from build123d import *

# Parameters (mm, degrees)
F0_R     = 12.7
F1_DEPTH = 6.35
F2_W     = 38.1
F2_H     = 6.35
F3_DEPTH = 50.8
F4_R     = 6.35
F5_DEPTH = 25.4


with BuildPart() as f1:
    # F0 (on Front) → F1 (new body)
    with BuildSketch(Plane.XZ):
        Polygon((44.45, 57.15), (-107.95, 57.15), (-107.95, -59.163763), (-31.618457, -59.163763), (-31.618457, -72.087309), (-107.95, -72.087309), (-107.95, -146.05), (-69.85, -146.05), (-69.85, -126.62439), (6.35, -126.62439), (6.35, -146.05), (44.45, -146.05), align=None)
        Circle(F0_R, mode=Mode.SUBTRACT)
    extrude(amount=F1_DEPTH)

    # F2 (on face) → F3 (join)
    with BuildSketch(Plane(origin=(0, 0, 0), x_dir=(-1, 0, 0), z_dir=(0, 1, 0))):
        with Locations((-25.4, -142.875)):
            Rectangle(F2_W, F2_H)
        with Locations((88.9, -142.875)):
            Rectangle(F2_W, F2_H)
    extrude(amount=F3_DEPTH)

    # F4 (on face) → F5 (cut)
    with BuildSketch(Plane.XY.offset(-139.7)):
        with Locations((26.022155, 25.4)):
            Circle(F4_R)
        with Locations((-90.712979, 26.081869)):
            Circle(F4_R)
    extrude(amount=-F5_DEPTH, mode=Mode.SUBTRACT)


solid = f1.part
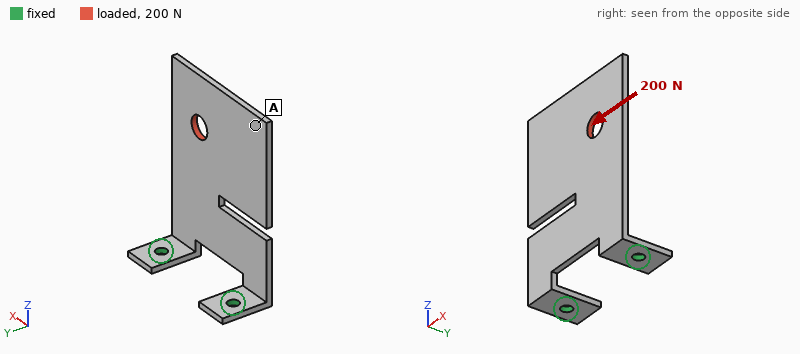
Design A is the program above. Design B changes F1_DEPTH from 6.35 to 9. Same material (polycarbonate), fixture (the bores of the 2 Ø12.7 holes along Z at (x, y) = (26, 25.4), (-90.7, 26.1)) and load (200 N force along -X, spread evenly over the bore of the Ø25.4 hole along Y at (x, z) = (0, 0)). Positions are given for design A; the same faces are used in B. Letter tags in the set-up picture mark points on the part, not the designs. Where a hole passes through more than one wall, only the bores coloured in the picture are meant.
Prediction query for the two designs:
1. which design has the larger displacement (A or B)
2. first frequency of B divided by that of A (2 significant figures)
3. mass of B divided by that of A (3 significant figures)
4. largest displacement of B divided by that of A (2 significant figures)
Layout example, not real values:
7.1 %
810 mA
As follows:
A
1.1
1.37
0.77
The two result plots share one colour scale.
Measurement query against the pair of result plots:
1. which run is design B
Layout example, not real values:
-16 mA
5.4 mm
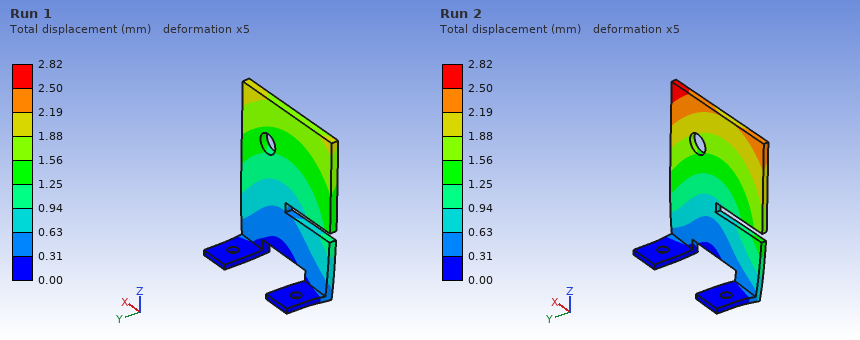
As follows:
Run 1
